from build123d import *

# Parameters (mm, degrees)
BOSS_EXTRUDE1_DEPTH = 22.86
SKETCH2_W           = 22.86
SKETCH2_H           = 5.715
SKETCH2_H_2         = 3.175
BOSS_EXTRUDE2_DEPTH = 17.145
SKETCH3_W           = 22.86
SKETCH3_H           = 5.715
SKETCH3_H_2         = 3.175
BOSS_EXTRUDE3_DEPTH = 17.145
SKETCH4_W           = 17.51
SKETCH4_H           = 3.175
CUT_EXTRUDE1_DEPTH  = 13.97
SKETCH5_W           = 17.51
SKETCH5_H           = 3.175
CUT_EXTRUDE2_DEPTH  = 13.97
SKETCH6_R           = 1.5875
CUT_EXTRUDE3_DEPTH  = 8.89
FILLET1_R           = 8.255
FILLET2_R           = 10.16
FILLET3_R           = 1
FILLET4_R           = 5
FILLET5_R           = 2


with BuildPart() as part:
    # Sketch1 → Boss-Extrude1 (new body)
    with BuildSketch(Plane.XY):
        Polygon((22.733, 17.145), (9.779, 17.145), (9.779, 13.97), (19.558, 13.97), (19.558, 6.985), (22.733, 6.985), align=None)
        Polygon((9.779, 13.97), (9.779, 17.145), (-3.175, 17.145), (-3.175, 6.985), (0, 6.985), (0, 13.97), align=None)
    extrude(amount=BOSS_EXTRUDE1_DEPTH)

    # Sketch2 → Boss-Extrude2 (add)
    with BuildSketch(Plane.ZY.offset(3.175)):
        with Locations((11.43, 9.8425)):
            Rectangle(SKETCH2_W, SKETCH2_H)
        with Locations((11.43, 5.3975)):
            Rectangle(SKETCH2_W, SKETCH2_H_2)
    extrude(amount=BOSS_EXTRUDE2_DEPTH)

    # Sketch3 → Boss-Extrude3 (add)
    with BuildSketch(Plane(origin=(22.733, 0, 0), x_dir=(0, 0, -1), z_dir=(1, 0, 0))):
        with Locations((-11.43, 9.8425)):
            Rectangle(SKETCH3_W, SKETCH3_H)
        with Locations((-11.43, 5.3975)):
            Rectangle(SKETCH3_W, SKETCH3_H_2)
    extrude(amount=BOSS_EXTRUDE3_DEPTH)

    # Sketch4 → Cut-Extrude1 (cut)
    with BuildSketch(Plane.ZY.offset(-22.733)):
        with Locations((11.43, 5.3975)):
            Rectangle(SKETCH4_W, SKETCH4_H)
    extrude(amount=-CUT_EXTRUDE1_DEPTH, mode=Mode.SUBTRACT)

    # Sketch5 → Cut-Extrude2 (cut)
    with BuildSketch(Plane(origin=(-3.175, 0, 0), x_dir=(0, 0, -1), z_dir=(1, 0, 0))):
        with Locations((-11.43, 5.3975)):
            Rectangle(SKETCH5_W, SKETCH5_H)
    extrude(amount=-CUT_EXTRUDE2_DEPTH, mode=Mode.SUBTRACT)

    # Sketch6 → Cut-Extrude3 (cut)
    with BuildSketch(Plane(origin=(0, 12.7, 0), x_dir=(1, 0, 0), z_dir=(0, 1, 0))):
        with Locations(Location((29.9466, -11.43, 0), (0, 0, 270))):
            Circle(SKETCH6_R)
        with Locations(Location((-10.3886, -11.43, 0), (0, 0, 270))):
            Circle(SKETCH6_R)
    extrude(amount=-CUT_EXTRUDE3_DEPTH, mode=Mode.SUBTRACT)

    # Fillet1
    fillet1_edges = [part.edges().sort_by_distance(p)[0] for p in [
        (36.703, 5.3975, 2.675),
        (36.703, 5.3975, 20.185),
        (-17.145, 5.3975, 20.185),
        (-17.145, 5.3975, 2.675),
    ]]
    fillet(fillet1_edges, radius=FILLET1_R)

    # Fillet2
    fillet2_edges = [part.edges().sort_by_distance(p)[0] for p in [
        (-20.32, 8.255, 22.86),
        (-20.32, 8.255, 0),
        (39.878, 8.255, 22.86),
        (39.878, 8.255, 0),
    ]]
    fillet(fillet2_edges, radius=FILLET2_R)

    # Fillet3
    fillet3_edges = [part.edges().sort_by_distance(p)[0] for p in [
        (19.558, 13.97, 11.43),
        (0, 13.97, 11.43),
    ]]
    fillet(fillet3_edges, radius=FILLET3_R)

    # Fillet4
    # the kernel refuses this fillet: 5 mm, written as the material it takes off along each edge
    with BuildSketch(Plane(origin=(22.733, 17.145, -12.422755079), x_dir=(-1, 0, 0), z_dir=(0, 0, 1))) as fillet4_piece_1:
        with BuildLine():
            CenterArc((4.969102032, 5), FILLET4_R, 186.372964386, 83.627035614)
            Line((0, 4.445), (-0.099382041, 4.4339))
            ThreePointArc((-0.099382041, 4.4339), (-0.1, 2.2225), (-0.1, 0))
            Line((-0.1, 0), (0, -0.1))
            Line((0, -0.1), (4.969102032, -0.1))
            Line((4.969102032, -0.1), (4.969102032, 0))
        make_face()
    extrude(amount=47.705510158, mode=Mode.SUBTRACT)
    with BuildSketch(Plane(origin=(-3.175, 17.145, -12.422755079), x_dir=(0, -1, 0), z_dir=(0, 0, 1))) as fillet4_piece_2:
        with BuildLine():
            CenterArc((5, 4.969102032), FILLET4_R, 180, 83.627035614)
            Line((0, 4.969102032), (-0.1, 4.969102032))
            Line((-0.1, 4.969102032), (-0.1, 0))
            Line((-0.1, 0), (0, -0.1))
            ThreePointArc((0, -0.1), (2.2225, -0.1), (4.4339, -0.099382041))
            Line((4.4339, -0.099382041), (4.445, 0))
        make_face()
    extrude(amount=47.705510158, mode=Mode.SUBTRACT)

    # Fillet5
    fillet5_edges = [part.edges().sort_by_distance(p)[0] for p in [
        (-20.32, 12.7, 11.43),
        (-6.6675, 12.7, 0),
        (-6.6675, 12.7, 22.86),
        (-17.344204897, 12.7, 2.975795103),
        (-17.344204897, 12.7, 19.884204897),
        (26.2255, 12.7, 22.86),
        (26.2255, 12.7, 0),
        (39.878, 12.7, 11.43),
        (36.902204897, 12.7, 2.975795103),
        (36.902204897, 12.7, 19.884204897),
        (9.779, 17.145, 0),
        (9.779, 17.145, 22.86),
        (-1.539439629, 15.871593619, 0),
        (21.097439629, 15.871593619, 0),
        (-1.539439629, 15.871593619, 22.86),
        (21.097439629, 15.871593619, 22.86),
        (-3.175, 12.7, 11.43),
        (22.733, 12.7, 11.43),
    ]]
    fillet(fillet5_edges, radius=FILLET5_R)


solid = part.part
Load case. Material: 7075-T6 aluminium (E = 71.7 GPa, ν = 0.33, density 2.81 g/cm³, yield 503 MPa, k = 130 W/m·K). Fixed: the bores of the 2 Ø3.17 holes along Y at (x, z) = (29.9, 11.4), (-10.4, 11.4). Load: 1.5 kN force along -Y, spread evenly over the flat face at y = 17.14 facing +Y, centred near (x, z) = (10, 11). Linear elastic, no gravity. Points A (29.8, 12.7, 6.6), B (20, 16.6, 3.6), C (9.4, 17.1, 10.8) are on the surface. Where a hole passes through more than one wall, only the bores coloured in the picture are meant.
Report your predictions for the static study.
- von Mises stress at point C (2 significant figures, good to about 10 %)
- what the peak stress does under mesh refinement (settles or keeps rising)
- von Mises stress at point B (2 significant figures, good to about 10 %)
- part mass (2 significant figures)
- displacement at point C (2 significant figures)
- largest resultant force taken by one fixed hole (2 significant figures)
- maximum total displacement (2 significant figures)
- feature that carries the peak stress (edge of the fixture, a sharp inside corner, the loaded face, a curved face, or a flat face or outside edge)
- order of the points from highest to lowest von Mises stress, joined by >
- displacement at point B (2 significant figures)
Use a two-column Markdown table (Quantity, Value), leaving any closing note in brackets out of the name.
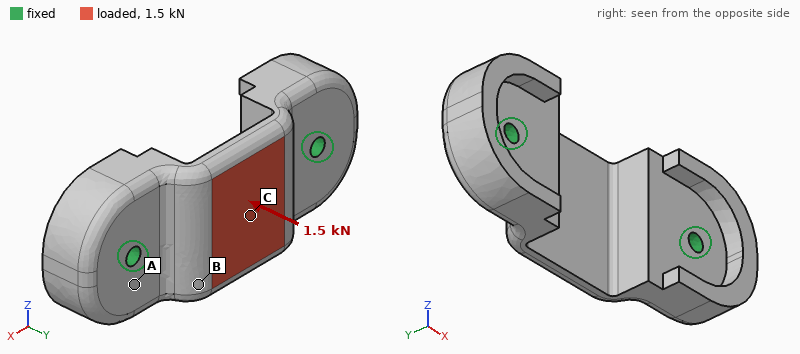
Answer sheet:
| Quantity | Value |
|---|---|
| von Mises stress at point C | 67 MPa |
| what the peak stress does under mesh refinement | keeps rising |
| von Mises stress at point B | 19 MPa |
| part mass | 20 g |
| displacement at point C | 27 µm |
| largest resultant force taken by one fixed hole | 1.3 kN |
| maximum total displacement | 28 µm |
| feature that carries the peak stress | edge of the fixture |
| order of the points from highest to lowest von Mises stress, joined by > | C > B > A |
| displacement at point B | 10 µm |
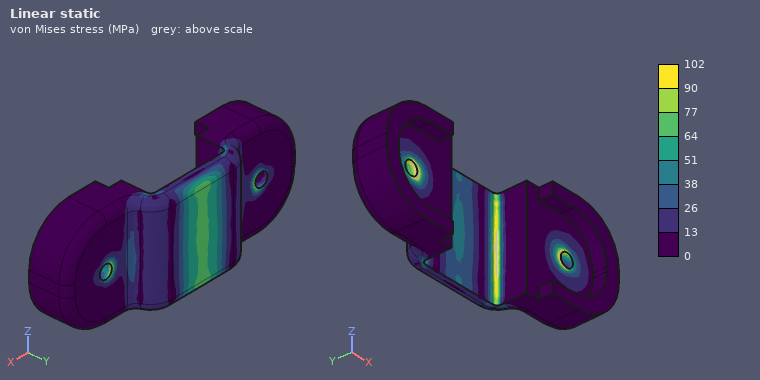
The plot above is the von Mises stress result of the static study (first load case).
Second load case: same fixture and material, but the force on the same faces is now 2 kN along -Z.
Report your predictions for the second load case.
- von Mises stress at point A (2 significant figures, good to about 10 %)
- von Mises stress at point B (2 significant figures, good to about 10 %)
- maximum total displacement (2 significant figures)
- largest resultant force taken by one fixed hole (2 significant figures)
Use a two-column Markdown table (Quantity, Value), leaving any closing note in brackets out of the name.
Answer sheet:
| Quantity | Value |
|---|---|
| von Mises stress at point A | 36 MPa |
| von Mises stress at point B | 44 MPa |
| maximum total displacement | 58 µm |
| largest resultant force taken by one fixed hole | 1.0 kN |
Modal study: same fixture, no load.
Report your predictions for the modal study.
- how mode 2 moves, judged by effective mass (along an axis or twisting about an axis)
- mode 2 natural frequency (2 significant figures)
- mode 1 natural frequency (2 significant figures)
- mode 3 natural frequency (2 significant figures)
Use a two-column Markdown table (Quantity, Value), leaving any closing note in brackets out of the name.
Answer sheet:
| Quantity | Value |
|---|---|
| how mode 2 moves, judged by effective mass | along Y |
| mode 2 natural frequency | 19 kHz |
| mode 1 natural frequency | 13 kHz |
| mode 3 natural frequency | 20 kHz |
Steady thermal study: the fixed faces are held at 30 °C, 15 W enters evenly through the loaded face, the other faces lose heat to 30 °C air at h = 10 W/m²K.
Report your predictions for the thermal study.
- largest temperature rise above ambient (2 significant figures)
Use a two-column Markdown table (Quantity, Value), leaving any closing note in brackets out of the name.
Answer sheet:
| Quantity | Value |
|---|---|
| largest temperature rise above ambient | 14 K |
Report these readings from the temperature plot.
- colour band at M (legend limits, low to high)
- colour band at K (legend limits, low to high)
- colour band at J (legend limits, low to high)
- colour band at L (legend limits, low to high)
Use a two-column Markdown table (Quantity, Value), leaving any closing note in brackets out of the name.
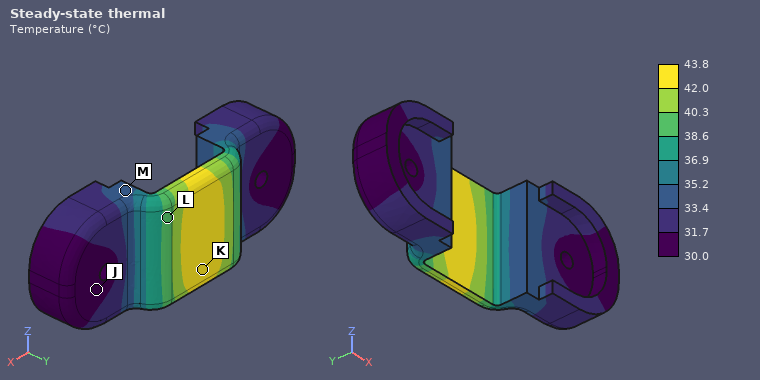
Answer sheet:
| Quantity | Value |
|---|---|
| colour band at M | 33.4 to 35.2 °C |
| colour band at K | 42.0 to 43.8 °C |
| colour band at J | 30.0 to 31.7 °C |
| colour band at L | 38.6 to 40.3 °C |
